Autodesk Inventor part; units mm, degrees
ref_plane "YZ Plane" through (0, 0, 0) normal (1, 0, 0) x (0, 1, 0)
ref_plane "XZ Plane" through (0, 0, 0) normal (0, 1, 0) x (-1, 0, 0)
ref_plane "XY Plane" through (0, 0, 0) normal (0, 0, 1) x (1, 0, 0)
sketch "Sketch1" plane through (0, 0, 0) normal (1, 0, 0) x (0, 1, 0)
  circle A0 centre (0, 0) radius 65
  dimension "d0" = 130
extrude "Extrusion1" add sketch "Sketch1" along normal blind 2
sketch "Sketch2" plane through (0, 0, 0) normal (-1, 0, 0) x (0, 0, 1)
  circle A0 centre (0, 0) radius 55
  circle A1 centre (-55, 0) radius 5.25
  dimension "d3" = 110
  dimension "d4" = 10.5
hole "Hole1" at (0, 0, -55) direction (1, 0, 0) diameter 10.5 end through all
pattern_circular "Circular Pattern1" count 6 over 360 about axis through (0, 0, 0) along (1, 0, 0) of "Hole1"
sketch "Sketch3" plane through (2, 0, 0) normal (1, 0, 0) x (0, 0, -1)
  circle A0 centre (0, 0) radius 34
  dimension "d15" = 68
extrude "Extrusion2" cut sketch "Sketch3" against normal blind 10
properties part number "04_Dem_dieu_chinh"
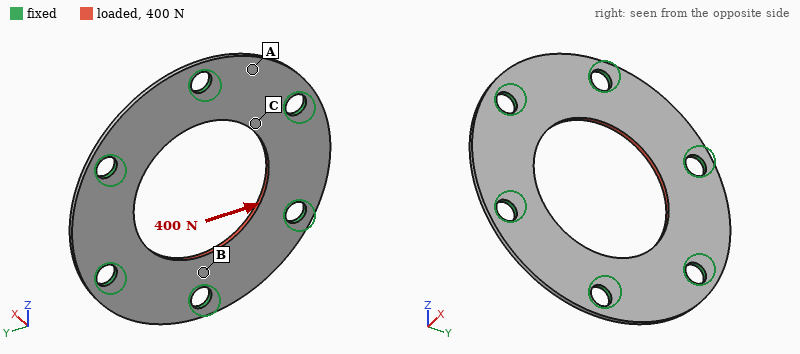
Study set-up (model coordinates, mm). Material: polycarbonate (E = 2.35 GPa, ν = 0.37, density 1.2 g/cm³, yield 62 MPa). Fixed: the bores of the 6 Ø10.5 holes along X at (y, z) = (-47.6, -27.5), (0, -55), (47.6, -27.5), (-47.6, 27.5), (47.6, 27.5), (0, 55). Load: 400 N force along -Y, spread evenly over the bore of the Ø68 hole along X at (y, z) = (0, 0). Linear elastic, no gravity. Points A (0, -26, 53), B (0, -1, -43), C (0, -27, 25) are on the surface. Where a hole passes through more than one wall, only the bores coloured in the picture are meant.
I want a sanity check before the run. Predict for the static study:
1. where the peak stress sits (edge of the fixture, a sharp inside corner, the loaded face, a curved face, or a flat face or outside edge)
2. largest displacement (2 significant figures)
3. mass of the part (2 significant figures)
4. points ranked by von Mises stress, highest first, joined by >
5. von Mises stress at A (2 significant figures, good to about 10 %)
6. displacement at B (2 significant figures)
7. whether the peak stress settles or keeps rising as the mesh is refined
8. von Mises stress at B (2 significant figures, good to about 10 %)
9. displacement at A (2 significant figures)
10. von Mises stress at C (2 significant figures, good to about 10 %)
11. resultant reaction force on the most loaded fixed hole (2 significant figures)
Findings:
edge of the fixture
19 µm
22 g
C > B > A
0.33 MPa
8.2 µm
keeps rising
0.87 MPa
6.7 µm
1.5 MPa
78 N
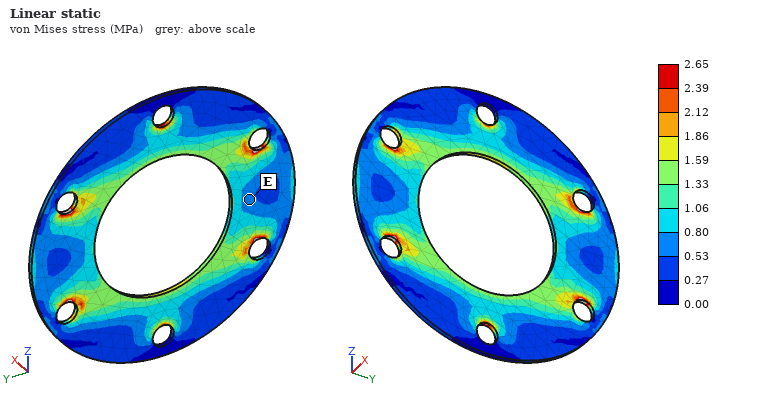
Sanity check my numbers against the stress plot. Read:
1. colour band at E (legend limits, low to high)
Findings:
0.53 to 0.80 MPa
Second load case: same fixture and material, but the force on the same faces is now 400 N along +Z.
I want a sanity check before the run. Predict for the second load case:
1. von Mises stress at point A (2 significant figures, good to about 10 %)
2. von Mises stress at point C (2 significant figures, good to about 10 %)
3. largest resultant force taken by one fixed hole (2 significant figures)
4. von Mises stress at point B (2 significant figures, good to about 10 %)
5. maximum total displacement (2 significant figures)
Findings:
0.48 MPa
0.79 MPa
86 N
1.7 MPa
19 µm
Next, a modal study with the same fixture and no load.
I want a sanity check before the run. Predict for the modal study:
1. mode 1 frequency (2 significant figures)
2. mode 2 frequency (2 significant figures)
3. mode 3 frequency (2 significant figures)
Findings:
1100 Hz
1100 Hz
1100 Hz
